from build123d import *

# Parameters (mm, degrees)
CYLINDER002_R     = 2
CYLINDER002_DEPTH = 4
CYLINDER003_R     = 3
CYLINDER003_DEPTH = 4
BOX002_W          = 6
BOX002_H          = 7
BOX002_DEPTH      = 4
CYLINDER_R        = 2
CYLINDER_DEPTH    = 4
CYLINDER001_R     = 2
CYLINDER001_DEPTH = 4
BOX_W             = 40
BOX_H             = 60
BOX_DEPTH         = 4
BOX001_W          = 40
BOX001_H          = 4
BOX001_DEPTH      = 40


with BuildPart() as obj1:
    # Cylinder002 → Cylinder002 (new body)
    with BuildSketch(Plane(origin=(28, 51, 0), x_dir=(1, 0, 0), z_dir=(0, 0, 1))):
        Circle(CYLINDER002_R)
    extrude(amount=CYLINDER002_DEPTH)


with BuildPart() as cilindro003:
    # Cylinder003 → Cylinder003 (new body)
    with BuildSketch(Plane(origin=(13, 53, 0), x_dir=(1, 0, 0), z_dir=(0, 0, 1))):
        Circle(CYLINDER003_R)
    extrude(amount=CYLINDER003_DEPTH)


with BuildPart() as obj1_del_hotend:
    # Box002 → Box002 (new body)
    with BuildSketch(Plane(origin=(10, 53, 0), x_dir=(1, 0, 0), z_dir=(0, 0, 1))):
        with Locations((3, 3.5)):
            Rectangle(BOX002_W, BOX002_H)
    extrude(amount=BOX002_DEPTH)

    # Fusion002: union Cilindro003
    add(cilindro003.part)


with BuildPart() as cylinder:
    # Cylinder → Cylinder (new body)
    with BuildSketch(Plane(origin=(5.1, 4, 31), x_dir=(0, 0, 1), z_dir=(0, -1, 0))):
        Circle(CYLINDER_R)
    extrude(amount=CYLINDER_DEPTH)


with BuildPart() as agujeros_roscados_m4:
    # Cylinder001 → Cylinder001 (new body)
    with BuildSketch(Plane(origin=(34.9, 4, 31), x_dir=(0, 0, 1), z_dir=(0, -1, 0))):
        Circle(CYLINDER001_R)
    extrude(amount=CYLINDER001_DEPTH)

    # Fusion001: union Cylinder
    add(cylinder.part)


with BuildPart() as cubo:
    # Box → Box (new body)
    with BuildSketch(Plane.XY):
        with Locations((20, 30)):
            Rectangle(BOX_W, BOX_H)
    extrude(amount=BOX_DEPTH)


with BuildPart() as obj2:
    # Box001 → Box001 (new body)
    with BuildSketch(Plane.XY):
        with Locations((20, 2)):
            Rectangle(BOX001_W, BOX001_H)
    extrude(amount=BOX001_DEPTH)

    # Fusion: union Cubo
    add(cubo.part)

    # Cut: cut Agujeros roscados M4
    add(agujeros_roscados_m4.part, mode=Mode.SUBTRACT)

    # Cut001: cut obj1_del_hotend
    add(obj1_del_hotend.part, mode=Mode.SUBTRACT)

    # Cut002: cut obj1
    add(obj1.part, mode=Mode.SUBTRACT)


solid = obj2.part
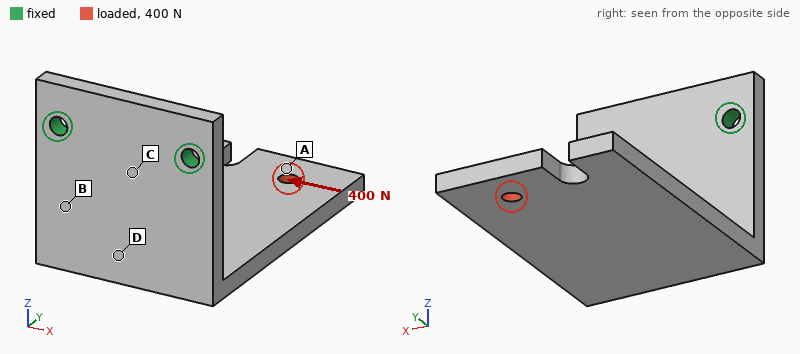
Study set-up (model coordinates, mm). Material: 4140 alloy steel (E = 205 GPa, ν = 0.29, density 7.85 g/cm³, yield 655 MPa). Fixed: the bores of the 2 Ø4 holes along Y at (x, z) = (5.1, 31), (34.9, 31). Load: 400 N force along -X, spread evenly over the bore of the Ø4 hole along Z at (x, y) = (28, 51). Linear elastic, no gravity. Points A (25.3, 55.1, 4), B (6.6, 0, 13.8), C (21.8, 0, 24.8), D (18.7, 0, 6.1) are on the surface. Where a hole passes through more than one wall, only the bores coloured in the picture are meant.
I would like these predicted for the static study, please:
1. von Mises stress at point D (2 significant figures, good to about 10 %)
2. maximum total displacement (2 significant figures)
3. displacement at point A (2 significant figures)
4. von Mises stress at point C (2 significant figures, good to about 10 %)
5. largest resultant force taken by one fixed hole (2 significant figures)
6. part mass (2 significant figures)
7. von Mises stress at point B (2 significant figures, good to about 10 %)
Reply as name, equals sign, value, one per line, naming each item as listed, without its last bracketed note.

von Mises stress at point D = 91 MPa
maximum total displacement = 0.29 mm
displacement at point A = 0.25 mm
von Mises stress at point C = 61 MPa
largest resultant force taken by one fixed hole = 760 N
part mass = 120 g
von Mises stress at point B = 110 MPa
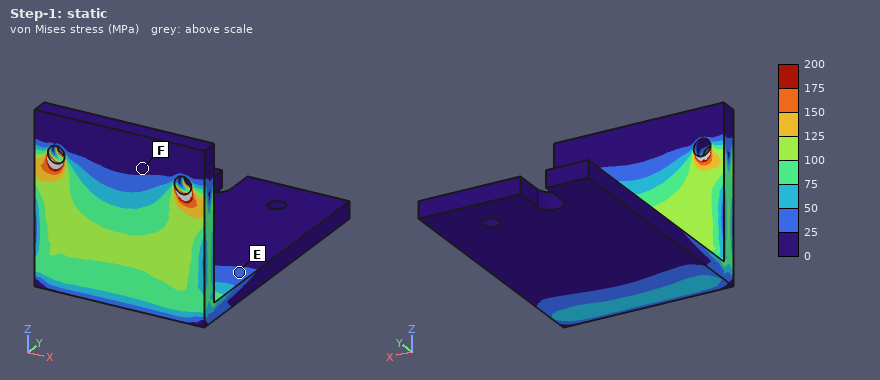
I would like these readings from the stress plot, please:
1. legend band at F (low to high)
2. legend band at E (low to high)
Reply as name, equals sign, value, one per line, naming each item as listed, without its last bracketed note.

legend band at F = 0 to 25 MPa
legend band at E = 25 to 50 MPa
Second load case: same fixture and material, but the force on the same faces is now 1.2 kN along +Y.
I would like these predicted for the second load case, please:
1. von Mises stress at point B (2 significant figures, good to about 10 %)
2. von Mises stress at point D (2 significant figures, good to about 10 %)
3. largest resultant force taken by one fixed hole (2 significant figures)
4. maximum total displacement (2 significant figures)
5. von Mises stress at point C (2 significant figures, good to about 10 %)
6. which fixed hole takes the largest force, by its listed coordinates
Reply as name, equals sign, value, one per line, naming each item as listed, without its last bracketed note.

von Mises stress at point B = 130 MPa
von Mises stress at point D = 70 MPa
largest resultant force taken by one fixed hole = 910 N
maximum total displacement = 0.78 mm
von Mises stress at point C = 180 MPa
which fixed hole takes the largest force, by its listed coordinates = (34.9, 31)
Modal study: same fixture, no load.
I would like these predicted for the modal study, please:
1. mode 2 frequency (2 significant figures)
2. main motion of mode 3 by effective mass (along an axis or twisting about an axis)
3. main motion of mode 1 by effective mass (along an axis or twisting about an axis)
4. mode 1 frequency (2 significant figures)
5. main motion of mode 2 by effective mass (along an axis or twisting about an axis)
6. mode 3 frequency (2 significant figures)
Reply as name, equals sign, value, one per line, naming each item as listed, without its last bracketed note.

mode 2 frequency = 1100 Hz
main motion of mode 3 by effective mass = along Y
main motion of mode 1 by effective mass = along Z
mode 1 frequency = 570 Hz
main motion of mode 2 by effective mass = along X
mode 3 frequency = 1900 Hz
